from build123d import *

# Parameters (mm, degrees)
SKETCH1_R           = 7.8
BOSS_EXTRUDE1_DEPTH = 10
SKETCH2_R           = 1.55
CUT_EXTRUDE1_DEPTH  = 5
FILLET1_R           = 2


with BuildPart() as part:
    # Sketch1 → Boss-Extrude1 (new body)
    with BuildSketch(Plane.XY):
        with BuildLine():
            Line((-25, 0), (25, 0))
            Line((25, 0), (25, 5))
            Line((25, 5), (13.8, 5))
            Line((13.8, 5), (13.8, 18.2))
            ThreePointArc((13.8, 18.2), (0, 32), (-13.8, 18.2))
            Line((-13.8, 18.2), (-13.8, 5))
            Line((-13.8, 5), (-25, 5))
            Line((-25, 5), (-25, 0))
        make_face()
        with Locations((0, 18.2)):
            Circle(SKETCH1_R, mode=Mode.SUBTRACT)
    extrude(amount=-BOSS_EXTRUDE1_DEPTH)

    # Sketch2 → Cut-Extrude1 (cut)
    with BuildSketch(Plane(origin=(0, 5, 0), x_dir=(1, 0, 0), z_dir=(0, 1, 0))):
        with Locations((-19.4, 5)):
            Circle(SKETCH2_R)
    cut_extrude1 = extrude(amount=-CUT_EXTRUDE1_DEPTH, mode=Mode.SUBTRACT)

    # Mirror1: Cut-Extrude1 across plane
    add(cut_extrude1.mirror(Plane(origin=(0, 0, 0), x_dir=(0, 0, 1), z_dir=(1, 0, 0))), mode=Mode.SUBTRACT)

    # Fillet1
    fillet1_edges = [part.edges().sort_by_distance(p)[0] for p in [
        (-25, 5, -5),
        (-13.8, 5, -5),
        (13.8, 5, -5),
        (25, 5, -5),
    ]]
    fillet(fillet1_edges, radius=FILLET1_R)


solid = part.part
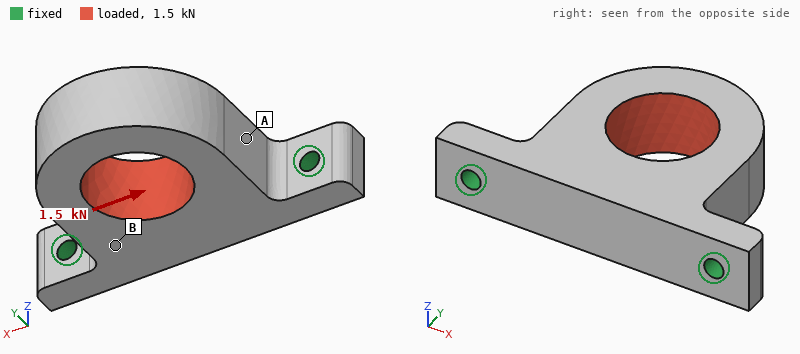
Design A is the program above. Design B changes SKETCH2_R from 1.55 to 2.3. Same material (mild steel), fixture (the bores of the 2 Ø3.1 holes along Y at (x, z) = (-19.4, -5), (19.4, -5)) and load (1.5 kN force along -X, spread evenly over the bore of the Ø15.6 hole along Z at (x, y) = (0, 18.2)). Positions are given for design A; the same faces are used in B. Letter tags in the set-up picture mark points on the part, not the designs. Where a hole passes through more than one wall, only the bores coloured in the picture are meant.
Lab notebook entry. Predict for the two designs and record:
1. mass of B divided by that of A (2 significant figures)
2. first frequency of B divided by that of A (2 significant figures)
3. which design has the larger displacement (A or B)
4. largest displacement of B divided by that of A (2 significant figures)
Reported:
0.99
1.1
A
0.92
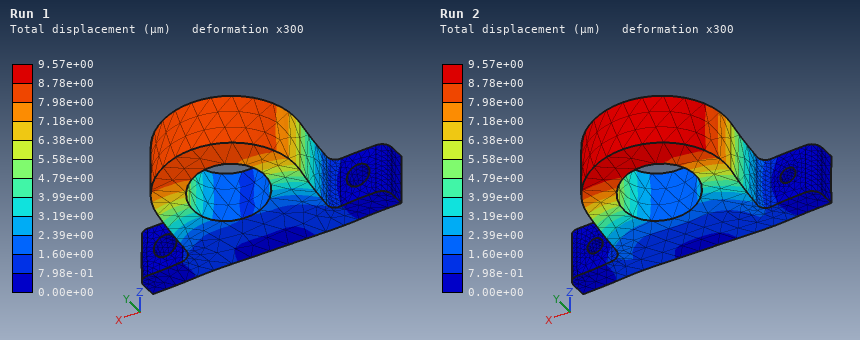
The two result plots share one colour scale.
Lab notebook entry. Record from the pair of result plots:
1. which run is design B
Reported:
Run 1
